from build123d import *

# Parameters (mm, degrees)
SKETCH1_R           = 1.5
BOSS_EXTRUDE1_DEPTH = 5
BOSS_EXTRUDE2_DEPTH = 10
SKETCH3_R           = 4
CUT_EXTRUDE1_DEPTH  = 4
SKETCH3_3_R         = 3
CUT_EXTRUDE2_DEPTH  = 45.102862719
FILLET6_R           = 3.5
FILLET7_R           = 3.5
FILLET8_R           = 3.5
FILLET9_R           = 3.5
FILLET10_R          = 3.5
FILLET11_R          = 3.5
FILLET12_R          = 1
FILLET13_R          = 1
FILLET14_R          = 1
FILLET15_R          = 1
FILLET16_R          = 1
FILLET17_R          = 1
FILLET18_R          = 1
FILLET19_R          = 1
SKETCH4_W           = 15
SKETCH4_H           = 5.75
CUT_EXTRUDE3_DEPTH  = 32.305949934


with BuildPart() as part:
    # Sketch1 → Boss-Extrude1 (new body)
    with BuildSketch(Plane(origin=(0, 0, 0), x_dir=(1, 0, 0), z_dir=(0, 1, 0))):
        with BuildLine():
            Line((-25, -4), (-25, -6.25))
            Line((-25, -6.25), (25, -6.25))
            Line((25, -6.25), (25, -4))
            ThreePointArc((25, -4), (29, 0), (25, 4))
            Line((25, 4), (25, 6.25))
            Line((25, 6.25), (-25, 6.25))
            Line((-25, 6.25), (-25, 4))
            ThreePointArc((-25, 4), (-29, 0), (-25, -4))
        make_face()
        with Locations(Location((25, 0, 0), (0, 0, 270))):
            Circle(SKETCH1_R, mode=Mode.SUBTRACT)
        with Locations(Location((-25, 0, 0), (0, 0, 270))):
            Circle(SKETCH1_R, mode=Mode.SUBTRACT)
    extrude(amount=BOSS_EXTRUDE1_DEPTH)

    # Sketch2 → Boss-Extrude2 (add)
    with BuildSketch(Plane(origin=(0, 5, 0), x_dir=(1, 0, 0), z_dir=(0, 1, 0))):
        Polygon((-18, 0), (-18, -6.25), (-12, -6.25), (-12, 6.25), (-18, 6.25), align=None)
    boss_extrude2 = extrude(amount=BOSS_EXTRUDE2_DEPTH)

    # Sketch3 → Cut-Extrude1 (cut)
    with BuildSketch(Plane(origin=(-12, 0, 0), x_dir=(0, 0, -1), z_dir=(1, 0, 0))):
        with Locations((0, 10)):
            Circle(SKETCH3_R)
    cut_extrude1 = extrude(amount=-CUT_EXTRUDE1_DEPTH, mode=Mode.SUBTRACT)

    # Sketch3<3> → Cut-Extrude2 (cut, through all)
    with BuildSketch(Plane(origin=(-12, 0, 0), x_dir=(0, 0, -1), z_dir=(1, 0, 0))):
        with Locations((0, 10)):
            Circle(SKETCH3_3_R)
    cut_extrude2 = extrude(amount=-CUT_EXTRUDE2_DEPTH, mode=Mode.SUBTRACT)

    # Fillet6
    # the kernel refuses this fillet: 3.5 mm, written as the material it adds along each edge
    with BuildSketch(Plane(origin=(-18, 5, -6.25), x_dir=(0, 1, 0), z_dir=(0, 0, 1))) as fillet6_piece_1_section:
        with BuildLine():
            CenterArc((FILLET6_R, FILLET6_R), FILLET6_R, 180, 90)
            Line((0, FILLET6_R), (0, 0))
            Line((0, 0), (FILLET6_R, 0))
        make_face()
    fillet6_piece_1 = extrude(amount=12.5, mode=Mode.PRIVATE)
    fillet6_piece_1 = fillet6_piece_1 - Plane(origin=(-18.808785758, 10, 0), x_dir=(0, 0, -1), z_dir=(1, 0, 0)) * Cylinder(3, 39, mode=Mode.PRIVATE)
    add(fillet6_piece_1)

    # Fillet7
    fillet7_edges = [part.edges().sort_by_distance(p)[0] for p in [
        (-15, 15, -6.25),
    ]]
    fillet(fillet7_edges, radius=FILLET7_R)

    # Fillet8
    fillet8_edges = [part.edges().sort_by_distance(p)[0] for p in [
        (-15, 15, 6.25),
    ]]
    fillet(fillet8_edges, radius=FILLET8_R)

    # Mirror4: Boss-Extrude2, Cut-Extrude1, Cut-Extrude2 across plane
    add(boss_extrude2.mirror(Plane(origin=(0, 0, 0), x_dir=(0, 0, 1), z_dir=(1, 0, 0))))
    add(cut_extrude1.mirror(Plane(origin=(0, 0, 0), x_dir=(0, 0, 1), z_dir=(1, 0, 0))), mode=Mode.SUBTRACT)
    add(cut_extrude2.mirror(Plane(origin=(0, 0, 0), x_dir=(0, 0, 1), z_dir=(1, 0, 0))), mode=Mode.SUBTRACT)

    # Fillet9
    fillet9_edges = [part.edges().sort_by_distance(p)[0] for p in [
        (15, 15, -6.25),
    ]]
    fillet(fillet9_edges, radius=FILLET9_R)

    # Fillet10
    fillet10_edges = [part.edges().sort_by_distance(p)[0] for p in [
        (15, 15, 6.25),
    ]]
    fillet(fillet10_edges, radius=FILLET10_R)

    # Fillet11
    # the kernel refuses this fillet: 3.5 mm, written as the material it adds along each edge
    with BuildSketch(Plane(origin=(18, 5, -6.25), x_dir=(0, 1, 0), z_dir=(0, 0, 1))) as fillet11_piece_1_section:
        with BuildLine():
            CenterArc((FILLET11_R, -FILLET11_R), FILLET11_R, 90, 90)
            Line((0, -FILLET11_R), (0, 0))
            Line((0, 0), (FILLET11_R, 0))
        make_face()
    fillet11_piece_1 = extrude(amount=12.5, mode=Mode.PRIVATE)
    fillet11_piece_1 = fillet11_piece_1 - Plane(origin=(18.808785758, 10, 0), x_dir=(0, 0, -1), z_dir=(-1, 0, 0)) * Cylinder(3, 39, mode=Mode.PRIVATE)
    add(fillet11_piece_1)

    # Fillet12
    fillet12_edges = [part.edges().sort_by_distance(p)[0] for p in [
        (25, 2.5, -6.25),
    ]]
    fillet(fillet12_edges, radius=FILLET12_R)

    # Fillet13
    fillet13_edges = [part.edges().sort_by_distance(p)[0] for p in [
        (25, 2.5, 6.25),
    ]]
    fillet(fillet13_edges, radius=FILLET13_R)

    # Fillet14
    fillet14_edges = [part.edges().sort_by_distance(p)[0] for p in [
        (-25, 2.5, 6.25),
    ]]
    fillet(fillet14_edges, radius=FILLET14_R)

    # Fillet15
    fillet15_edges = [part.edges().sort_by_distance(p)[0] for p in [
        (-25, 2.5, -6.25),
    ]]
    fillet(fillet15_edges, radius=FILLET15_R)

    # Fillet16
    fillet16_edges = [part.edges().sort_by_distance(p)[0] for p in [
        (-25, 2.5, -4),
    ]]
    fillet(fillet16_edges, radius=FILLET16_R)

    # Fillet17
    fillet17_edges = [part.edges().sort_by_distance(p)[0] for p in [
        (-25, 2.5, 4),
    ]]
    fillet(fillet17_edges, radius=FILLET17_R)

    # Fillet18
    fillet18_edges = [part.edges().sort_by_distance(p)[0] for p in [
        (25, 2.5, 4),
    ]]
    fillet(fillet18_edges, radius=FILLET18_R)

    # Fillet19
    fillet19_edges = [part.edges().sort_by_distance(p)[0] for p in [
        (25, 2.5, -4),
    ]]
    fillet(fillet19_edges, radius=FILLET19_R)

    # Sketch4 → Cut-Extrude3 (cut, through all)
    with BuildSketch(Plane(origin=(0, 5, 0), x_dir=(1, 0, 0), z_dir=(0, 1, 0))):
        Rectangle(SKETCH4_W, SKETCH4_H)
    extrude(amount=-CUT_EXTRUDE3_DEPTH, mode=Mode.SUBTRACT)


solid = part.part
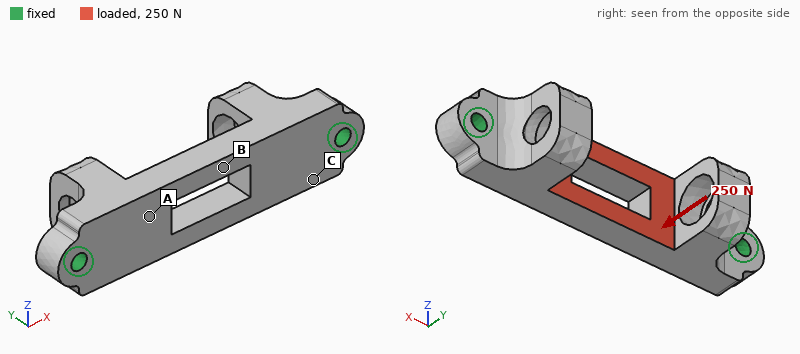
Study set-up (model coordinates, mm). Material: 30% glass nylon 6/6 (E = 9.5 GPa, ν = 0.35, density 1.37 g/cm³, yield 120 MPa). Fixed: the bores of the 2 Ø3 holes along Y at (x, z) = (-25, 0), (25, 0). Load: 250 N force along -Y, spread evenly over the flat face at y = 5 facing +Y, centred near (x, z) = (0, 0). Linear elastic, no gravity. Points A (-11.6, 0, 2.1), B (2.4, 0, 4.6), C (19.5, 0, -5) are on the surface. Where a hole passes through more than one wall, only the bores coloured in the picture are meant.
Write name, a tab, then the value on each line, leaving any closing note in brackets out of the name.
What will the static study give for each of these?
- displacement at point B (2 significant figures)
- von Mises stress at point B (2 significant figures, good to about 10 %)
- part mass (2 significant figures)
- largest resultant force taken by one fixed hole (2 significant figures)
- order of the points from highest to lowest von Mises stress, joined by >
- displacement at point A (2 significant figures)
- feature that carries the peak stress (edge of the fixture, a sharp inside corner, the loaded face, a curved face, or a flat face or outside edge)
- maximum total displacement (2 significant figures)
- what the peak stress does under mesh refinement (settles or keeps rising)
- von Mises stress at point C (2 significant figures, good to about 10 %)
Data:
displacement at point B	0.14 mm
von Mises stress at point B	23 MPa
part mass	5.3 g
largest resultant force taken by one fixed hole	130 N
order of the points from highest to lowest von Mises stress, joined by >	B > C > A
displacement at point A	0.089 mm
feature that carries the peak stress	edge of the fixture
maximum total displacement	0.15 mm
what the peak stress does under mesh refinement	keeps rising
von Mises stress at point C	13 MPa
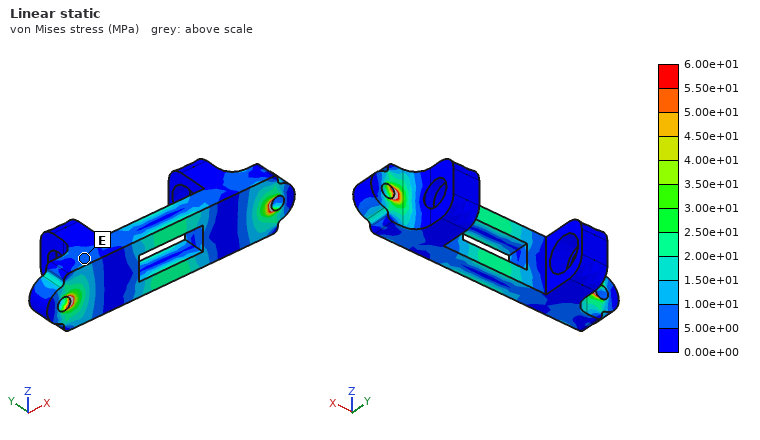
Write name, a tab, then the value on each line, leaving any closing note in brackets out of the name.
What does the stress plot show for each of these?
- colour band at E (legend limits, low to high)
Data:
colour band at E	5.00e+00 to 1.00e+01 MPa
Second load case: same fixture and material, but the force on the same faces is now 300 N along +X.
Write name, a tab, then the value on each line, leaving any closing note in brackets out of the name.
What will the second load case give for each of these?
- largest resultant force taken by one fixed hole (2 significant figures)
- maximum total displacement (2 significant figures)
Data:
largest resultant force taken by one fixed hole	150 N
maximum total displacement	7.4 µm
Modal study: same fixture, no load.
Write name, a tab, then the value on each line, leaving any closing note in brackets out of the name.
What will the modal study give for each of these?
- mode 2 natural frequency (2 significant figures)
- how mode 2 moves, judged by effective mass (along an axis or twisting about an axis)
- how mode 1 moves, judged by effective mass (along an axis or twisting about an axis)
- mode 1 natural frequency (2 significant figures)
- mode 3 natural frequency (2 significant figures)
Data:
mode 2 natural frequency	6800 Hz
how mode 2 moves, judged by effective mass	along Z
how mode 1 moves, judged by effective mass	along Y
mode 1 natural frequency	4600 Hz
mode 3 natural frequency	8000 Hz
